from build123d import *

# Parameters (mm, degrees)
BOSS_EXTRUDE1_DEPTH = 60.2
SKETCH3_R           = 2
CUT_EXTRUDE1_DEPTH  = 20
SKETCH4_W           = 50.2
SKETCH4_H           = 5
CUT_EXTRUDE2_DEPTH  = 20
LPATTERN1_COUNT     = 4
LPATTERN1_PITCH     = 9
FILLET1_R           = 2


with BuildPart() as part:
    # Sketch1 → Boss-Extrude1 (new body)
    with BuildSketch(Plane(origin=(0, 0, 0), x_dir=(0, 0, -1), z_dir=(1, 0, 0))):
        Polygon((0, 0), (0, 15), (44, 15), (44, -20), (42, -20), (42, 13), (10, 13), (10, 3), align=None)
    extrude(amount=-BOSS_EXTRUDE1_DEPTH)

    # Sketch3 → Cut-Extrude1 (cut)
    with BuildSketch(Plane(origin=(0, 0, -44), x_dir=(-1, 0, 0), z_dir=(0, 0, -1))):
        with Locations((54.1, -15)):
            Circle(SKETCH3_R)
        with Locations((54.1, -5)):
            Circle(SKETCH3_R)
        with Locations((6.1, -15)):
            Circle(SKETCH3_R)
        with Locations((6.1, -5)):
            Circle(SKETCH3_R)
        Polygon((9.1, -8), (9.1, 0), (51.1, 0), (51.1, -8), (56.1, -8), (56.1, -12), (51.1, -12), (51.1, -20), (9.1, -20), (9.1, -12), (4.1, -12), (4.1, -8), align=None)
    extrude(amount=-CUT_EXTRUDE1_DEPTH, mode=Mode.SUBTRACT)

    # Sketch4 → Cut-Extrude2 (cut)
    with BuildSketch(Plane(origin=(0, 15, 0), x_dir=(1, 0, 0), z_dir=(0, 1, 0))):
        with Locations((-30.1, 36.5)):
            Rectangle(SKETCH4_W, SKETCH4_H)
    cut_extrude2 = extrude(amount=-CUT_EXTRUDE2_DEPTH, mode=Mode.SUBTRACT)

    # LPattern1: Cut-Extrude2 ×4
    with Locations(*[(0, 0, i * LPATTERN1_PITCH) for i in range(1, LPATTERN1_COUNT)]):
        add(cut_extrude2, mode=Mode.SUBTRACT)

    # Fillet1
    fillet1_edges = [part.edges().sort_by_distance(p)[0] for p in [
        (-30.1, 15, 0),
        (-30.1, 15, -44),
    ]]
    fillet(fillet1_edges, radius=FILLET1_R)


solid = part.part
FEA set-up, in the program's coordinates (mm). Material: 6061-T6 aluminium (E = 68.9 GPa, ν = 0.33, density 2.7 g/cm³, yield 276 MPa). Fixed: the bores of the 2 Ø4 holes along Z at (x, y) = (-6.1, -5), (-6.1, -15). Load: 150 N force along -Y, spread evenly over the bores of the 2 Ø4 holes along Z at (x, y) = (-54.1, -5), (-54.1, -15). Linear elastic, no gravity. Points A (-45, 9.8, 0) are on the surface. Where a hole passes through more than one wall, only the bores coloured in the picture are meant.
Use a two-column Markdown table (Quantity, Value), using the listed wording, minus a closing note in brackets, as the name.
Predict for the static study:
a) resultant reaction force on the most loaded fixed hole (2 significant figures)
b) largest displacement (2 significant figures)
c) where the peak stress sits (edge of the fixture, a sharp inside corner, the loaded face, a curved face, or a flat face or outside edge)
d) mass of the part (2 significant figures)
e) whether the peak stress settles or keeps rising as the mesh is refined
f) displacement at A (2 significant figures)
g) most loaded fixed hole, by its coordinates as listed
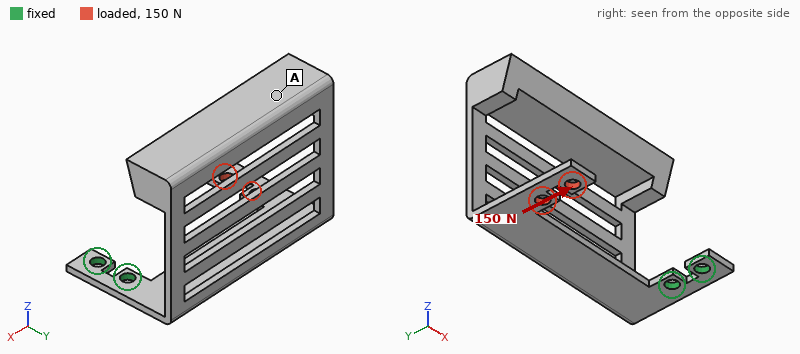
| Quantity | Value |
|---|---|
| resultant reaction force on the most loaded fixed hole | 510 N |
| largest displacement | 0.70 mm |
| where the peak stress sits | a sharp inside corner |
| mass of the part | 29 g |
| whether the peak stress settles or keeps rising as the mesh is refined | keeps rising |
| displacement at A | 0.46 mm |
| most loaded fixed hole, by its coordinates as listed | (-6.1, -5) |
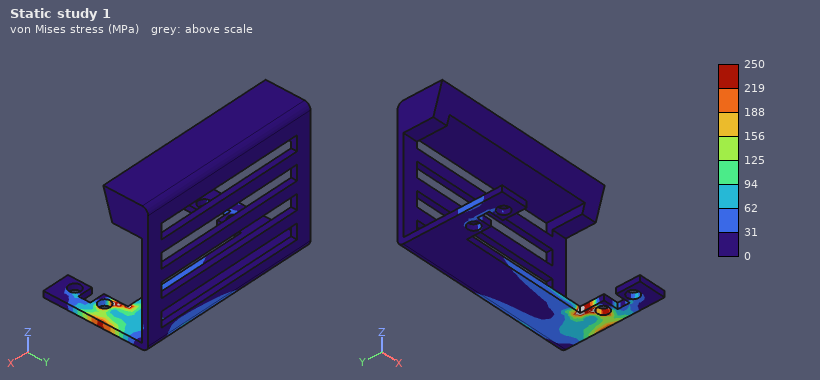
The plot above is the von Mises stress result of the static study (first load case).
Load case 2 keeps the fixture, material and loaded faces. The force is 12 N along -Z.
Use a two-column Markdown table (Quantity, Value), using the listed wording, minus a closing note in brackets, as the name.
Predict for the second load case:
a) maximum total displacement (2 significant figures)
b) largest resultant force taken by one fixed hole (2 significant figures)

| Quantity | Value |
|---|---|
| maximum total displacement | 0.92 mm |
| largest resultant force taken by one fixed hole | 6.0 N |
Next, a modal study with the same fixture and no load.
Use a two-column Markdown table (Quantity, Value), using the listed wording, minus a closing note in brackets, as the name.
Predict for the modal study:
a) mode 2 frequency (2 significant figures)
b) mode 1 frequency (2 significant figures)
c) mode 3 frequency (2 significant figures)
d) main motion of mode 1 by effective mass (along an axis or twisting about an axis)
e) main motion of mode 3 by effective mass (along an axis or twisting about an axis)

| Quantity | Value |
|---|---|
| mode 2 frequency | 150 Hz |
| mode 1 frequency | 120 Hz |
| mode 3 frequency | 580 Hz |
| main motion of mode 1 by effective mass | along Y |
| main motion of mode 3 by effective mass | along Z |
